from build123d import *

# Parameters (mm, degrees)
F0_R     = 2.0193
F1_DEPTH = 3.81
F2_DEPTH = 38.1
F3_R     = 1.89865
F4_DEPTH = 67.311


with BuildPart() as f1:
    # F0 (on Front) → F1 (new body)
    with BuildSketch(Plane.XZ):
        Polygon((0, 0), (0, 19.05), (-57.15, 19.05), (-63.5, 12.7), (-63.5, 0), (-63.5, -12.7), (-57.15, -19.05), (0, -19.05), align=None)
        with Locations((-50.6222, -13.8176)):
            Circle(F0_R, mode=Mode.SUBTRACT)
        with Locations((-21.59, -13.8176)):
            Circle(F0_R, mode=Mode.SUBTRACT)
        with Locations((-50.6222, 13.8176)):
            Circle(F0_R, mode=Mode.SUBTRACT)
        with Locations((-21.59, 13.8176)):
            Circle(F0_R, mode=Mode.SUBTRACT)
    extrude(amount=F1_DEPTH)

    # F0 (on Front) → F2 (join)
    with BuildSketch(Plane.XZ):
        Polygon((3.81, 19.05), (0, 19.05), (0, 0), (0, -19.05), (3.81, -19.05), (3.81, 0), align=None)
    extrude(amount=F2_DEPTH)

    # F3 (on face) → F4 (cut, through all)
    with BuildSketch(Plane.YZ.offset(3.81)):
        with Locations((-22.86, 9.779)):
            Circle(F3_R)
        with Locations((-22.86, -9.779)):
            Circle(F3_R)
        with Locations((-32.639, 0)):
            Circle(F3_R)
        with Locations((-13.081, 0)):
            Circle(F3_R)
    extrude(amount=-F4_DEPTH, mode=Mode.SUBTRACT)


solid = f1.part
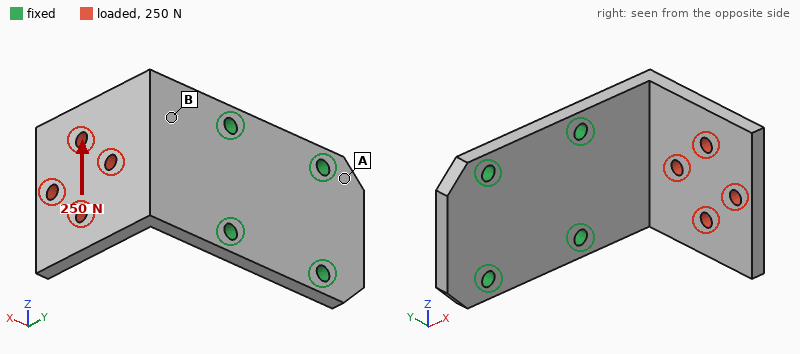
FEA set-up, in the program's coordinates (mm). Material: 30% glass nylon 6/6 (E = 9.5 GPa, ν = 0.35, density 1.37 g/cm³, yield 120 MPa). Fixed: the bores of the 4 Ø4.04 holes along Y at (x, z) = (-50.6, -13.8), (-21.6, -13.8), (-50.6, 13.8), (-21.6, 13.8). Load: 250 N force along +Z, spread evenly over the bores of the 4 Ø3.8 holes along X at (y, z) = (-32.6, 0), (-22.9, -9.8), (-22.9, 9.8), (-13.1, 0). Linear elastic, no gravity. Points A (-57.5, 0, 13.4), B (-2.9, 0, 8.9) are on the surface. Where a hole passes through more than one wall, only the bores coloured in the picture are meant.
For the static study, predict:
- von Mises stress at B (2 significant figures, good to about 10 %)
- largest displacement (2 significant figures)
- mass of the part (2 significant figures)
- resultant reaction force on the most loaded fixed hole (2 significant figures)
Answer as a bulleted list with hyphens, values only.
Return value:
- 24 MPa
- 0.98 mm
- 19 g
- 290 N
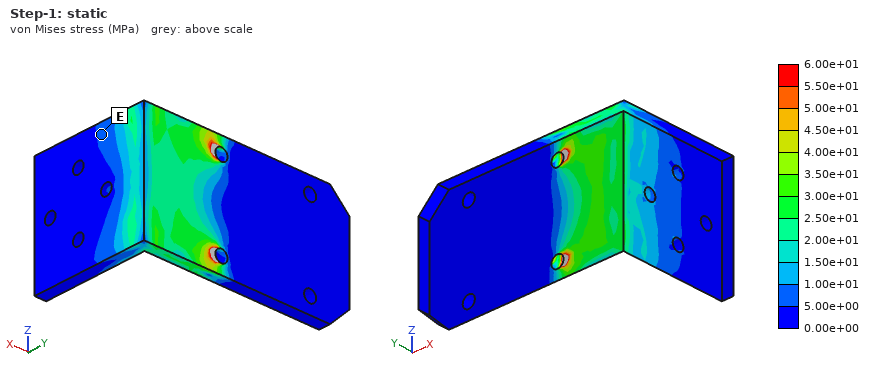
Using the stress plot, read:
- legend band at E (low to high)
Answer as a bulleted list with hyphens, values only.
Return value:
- 5.00e+00 to 1.00e+01 MPa
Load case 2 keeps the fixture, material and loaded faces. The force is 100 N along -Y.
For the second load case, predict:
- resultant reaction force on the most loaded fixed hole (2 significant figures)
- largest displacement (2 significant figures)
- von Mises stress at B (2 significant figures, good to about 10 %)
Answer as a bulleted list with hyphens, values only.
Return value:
- 58 N
- 0.65 mm
- 5.3 MPa
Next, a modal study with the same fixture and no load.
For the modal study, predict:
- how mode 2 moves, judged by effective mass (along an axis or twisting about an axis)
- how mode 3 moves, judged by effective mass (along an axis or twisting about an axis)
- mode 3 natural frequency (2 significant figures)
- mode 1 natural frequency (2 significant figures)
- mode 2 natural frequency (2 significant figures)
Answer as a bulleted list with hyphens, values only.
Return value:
- along Z
- along Y
- 1800 Hz
- 620 Hz
- 1200 Hz
